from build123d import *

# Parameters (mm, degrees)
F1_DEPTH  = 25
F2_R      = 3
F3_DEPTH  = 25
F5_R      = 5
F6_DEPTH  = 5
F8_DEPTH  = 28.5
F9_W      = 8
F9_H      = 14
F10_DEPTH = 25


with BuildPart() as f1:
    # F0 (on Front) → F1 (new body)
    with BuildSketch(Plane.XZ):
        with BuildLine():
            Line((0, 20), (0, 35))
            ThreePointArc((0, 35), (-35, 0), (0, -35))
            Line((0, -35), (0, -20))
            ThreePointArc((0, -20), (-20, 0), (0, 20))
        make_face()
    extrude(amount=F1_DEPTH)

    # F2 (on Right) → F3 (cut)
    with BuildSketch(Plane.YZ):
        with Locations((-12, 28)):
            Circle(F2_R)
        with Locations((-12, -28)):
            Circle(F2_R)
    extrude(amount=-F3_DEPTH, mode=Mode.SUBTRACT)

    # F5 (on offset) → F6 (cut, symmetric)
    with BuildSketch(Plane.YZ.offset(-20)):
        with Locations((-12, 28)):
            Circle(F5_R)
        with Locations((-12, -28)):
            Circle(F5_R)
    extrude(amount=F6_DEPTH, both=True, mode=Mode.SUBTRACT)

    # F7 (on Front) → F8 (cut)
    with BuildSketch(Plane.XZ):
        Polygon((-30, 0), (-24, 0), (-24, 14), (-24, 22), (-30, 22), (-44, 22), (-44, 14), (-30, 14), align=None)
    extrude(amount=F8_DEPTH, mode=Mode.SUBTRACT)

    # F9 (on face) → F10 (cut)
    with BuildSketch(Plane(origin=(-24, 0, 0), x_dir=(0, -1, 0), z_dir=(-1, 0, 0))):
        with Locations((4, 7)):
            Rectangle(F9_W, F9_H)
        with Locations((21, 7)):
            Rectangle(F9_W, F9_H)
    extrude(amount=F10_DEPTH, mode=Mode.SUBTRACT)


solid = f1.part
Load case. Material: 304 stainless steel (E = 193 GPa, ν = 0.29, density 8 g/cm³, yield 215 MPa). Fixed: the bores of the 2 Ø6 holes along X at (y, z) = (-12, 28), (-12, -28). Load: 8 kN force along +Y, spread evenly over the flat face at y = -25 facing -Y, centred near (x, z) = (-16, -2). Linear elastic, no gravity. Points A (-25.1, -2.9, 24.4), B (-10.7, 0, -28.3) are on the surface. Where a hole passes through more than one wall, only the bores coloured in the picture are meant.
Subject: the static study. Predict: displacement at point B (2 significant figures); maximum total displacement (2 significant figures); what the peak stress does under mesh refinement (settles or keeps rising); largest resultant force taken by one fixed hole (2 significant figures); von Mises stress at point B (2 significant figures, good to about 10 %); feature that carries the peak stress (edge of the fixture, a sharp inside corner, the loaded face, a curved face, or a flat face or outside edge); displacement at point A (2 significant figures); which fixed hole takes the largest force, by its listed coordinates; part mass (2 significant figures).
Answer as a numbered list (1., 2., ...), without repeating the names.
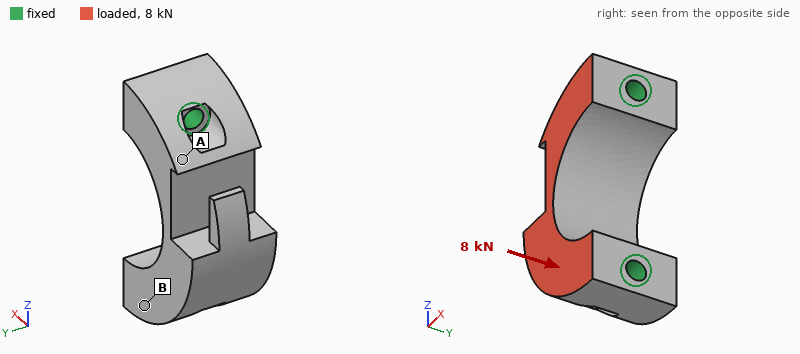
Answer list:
1. 2.8 µm
2. 15 µm
3. keeps rising
4. 4.3 kN
5. 25 MPa
6. edge of the fixture
7. 4.3 µm
8. (-12, -28)
9. 210 g
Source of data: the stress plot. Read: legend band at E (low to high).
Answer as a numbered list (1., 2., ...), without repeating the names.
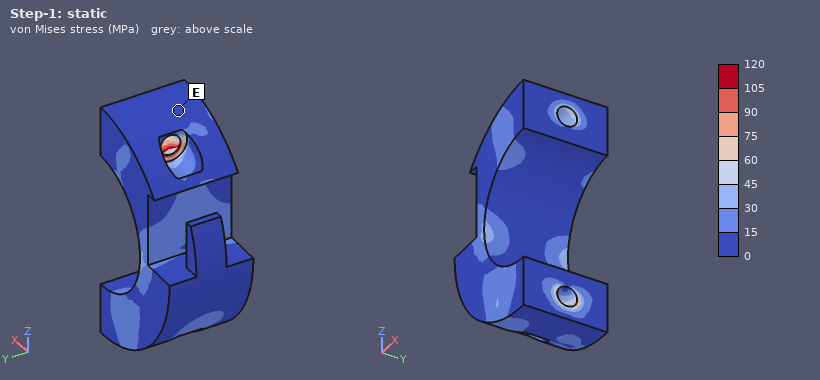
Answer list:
1. 0 to 15 MPa
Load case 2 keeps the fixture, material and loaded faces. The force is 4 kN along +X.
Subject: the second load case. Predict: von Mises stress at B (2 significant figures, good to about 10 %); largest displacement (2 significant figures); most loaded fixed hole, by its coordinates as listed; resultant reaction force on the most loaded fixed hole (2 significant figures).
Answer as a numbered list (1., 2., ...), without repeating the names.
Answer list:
1. 13 MPa
2. 9.4 µm
3. (-12, -28)
4. 2.3 kN
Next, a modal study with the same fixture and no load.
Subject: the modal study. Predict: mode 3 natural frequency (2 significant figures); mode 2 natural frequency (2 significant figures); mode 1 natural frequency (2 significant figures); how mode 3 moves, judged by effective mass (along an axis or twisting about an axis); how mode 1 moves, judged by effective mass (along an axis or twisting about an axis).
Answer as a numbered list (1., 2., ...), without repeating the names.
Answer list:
1. 18 kHz
2. 13 kHz
3. 9800 Hz
4. along Z
5. along Y
